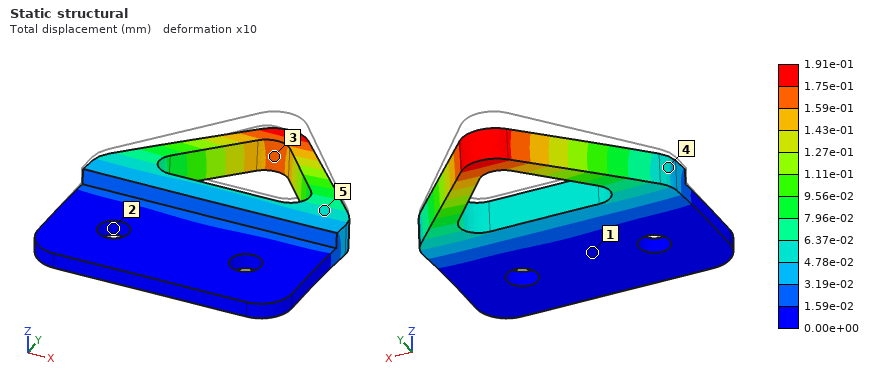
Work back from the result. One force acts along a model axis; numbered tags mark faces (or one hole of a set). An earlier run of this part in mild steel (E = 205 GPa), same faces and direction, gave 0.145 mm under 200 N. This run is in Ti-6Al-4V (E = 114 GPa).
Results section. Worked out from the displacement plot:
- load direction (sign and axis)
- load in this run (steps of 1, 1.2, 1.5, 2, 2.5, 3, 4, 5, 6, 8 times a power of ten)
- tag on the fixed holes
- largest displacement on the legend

-Z
150 N
2
1.91e-01 mm
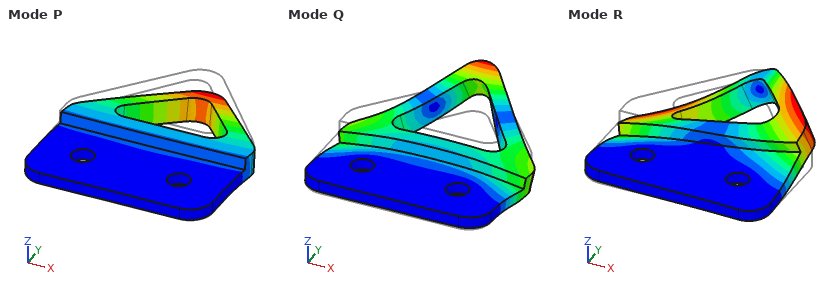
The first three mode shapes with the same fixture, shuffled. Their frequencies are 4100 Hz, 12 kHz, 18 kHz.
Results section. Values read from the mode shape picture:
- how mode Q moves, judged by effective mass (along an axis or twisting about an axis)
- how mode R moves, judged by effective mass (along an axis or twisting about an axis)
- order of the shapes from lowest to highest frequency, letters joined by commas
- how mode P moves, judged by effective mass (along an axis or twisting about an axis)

along Z
twisting about Y
P, R, Q
along Z
